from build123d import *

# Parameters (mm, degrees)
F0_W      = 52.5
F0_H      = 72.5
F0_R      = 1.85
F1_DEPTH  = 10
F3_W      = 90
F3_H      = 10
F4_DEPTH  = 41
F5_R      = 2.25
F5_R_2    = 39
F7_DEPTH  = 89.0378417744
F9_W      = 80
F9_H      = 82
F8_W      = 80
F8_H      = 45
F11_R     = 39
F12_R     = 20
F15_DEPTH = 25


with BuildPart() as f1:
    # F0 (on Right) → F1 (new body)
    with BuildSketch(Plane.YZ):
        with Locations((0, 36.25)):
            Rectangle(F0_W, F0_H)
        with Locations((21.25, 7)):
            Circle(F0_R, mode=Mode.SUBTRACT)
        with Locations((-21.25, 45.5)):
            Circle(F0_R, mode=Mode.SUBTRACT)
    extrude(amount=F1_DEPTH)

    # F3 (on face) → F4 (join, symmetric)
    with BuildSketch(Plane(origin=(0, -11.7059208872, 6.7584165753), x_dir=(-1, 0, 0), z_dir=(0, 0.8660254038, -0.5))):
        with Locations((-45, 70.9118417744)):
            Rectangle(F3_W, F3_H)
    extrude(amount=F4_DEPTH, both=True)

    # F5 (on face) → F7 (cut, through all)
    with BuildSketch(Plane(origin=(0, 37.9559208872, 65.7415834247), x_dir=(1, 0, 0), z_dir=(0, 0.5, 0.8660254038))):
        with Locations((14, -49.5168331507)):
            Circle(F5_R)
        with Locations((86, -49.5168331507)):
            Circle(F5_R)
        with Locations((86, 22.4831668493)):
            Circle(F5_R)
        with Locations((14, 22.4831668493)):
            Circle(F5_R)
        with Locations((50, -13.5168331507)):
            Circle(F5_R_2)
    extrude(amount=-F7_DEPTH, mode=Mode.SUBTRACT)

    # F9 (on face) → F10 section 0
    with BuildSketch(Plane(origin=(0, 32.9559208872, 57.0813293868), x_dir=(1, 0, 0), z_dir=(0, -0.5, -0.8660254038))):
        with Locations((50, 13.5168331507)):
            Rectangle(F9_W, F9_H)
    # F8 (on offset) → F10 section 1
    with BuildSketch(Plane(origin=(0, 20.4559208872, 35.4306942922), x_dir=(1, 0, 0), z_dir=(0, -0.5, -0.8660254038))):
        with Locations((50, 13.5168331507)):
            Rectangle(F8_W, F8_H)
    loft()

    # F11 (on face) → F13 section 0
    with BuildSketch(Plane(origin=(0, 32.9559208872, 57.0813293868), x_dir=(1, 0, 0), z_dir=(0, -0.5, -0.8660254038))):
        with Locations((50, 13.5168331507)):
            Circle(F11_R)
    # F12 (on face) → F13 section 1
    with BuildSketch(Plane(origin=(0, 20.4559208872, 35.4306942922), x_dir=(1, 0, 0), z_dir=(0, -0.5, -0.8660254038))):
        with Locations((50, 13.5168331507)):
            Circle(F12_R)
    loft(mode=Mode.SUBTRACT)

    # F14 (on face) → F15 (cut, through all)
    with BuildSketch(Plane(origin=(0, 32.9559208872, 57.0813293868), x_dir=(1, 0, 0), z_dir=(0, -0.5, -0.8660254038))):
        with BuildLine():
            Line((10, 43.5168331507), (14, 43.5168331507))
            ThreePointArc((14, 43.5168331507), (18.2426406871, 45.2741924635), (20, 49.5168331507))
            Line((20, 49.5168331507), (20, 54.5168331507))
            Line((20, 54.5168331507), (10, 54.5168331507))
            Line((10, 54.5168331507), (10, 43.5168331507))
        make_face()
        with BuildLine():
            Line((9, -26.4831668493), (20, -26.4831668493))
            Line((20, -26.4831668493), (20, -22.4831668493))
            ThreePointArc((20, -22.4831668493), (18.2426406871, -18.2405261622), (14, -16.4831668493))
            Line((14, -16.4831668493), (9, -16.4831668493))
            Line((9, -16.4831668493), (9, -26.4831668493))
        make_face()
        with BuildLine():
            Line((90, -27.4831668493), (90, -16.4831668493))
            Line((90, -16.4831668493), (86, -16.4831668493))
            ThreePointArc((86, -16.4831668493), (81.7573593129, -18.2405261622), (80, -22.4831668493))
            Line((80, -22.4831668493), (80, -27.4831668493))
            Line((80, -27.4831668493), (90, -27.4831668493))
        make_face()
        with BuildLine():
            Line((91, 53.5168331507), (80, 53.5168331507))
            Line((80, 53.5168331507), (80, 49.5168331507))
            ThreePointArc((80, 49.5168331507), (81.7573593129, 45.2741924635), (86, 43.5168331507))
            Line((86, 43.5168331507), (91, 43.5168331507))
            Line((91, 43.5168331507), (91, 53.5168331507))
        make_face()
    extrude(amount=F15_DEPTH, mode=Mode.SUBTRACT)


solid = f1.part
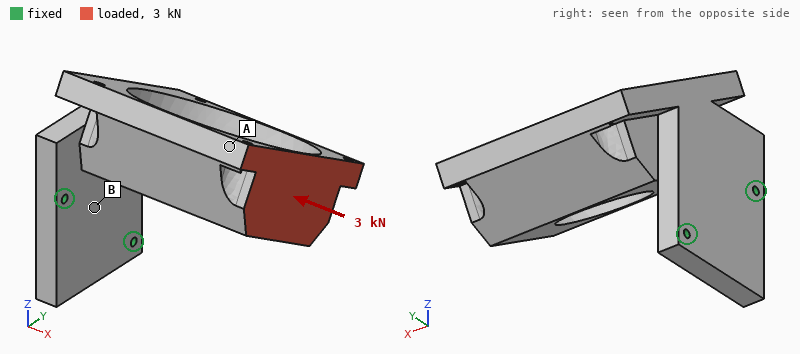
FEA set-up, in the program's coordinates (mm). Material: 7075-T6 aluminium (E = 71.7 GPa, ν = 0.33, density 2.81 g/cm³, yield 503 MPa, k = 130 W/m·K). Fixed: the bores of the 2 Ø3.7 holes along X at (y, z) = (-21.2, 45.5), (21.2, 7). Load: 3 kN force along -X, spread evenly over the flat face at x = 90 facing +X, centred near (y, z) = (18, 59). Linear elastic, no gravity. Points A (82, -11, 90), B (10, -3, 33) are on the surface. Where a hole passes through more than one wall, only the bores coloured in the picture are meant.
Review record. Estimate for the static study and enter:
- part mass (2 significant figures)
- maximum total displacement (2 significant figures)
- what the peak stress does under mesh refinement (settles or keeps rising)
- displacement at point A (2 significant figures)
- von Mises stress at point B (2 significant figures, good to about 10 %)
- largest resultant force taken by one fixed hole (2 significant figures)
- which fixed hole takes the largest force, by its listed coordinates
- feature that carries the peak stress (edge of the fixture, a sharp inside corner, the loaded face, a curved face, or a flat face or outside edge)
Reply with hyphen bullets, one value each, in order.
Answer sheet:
- 320 g
- 0.84 mm
- keeps rising
- 0.64 mm
- 43 MPa
- 1.8 kN
- (-21.2, 45.5)
- edge of the fixture
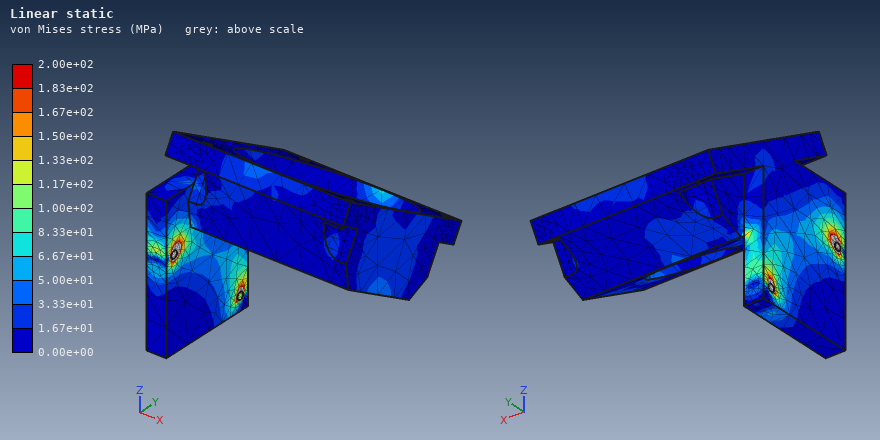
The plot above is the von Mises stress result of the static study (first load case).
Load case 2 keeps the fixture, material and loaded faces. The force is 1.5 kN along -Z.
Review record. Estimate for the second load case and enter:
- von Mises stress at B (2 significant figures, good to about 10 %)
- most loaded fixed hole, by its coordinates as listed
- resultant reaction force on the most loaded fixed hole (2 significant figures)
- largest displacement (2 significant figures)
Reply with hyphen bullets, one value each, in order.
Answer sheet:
- 53 MPa
- (21.2, 7)
- 1.8 kN
- 1.0 mm
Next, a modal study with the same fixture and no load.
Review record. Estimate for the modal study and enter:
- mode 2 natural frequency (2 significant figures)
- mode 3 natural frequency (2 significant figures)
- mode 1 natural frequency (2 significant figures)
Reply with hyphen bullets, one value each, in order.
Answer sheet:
- 1000 Hz
- 2100 Hz
- 580 Hz
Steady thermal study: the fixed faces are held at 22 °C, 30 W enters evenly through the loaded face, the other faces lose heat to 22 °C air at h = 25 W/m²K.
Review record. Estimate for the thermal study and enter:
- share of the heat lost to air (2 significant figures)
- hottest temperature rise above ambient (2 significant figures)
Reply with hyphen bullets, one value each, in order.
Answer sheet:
- 45 %
- 46 K
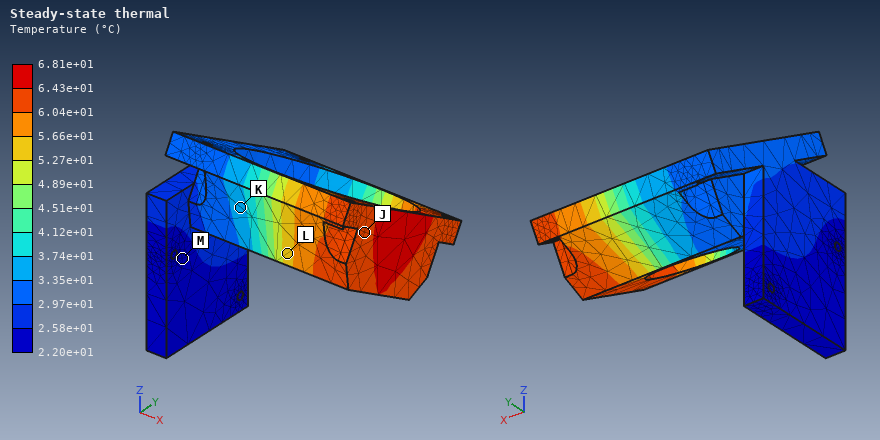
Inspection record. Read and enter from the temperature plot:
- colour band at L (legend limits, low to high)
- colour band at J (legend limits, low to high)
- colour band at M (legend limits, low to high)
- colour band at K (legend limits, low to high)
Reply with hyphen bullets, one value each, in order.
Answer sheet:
- 5.27e+01 to 5.66e+01 °C
- 6.04e+01 to 6.43e+01 °C
- 2.20e+01 to 2.58e+01 °C
- 3.35e+01 to 3.74e+01 °C
